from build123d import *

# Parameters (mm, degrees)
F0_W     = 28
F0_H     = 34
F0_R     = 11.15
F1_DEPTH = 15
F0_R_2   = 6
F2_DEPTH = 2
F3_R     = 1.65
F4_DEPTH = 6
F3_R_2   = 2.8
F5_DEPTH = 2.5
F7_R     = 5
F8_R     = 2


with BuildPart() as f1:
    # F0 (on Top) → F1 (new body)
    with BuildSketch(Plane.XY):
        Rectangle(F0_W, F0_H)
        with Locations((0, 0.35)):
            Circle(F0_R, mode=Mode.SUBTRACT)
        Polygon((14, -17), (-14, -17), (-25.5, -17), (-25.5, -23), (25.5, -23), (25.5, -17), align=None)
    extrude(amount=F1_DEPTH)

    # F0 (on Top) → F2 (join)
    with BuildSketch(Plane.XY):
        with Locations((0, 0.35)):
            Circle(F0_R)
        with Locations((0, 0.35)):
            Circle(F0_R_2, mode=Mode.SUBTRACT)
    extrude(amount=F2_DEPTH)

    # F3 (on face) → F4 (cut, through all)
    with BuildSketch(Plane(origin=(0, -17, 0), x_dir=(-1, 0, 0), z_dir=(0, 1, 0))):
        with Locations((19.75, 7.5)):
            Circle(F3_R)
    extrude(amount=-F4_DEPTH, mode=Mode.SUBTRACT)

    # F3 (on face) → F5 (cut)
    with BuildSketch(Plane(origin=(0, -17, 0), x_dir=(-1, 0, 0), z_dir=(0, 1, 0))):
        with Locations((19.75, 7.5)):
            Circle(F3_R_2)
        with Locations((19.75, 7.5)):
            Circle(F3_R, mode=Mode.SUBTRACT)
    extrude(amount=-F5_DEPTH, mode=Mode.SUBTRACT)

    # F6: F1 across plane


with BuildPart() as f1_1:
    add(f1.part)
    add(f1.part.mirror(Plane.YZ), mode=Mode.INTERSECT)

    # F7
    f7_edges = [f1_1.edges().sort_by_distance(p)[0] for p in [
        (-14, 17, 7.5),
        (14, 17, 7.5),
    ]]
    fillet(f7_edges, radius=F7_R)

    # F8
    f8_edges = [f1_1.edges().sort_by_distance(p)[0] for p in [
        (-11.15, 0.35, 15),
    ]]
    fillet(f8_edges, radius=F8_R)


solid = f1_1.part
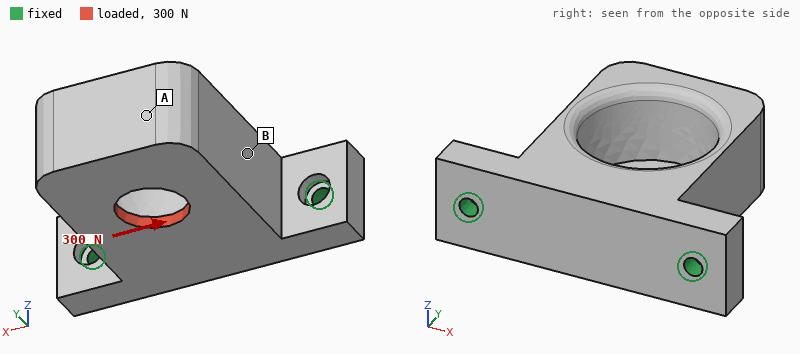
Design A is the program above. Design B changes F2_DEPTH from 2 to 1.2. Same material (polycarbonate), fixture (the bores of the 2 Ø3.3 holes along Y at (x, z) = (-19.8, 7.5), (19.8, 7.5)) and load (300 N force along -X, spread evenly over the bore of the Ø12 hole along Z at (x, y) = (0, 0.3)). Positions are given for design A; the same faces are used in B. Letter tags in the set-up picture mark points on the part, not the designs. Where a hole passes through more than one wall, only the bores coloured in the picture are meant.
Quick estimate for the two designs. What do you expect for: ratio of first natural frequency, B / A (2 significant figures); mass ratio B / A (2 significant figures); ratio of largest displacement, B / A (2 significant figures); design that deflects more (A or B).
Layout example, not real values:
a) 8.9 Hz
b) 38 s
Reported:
a) 1.0
b) 0.98
c) 1.1
d) B
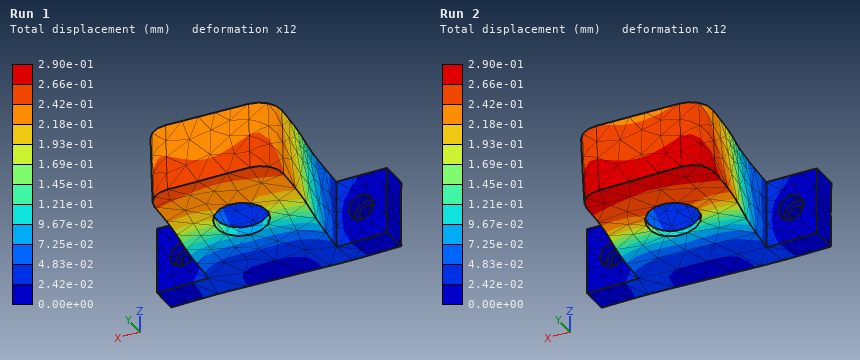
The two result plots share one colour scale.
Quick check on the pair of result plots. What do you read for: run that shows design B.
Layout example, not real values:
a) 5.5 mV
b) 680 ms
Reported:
a) Run 2
